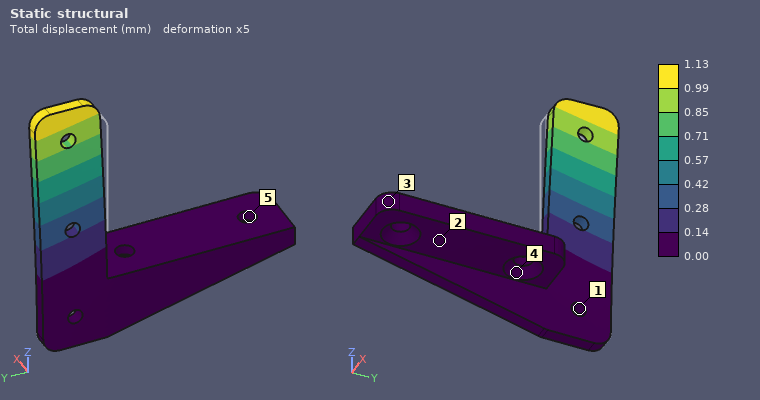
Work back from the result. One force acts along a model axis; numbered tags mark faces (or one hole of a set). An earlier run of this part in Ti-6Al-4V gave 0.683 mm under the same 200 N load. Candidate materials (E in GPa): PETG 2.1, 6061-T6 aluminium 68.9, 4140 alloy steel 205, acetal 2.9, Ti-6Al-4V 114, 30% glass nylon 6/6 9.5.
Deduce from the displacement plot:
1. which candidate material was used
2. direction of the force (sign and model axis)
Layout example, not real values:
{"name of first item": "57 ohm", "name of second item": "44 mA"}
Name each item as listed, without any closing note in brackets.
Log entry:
{"which candidate material was used": "6061-T6 aluminium", "direction of the force": "+X"}
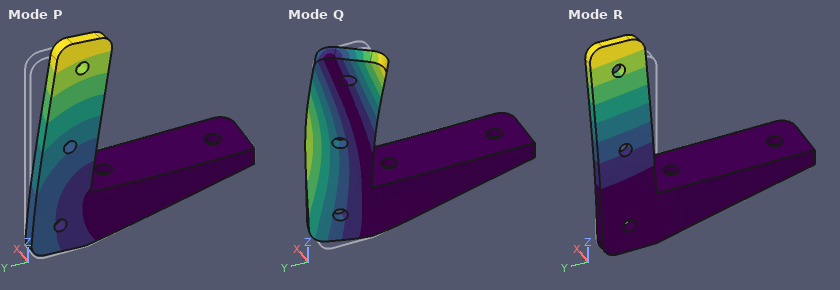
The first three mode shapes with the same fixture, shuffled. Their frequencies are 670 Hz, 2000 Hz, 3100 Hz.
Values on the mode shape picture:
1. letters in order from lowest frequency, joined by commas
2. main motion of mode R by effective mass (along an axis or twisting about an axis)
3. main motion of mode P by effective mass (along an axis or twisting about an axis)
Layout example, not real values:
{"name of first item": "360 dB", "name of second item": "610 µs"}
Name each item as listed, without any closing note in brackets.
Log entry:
{"letters in order from lowest frequency, joined by commas": "R, P, Q", "main motion of mode R by effective mass": "along X", "main motion of mode P by effective mass": "along Y"}
